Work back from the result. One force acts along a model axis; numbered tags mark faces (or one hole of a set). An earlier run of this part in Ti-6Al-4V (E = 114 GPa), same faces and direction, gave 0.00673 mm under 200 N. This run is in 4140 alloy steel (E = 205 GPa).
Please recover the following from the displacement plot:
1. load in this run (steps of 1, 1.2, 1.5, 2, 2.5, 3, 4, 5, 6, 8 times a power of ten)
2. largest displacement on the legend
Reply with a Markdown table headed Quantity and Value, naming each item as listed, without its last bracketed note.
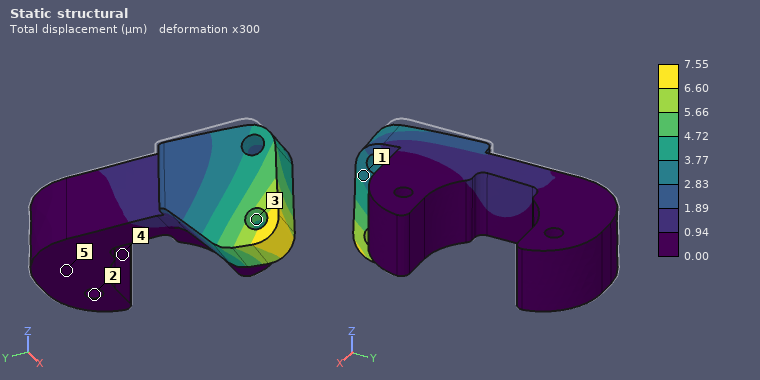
| Quantity | Value |
|---|---|
| load in this run | 400 N |
| largest displacement on the legend | 7.55 µm |
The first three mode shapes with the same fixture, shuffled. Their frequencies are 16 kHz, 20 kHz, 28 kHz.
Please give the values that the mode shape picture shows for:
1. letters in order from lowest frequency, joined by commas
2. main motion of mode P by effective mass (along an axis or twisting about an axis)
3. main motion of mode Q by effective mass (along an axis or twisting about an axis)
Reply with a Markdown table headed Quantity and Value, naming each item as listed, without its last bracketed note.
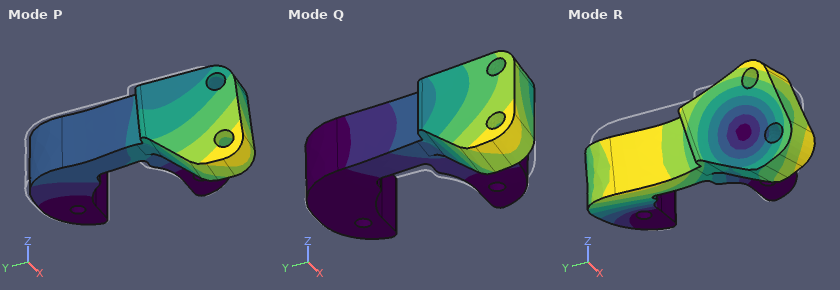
| Quantity | Value |
|---|---|
| letters in order from lowest frequency, joined by commas | Q, P, R |
| main motion of mode P by effective mass | along Y |
| main motion of mode Q by effective mass | along Z |
